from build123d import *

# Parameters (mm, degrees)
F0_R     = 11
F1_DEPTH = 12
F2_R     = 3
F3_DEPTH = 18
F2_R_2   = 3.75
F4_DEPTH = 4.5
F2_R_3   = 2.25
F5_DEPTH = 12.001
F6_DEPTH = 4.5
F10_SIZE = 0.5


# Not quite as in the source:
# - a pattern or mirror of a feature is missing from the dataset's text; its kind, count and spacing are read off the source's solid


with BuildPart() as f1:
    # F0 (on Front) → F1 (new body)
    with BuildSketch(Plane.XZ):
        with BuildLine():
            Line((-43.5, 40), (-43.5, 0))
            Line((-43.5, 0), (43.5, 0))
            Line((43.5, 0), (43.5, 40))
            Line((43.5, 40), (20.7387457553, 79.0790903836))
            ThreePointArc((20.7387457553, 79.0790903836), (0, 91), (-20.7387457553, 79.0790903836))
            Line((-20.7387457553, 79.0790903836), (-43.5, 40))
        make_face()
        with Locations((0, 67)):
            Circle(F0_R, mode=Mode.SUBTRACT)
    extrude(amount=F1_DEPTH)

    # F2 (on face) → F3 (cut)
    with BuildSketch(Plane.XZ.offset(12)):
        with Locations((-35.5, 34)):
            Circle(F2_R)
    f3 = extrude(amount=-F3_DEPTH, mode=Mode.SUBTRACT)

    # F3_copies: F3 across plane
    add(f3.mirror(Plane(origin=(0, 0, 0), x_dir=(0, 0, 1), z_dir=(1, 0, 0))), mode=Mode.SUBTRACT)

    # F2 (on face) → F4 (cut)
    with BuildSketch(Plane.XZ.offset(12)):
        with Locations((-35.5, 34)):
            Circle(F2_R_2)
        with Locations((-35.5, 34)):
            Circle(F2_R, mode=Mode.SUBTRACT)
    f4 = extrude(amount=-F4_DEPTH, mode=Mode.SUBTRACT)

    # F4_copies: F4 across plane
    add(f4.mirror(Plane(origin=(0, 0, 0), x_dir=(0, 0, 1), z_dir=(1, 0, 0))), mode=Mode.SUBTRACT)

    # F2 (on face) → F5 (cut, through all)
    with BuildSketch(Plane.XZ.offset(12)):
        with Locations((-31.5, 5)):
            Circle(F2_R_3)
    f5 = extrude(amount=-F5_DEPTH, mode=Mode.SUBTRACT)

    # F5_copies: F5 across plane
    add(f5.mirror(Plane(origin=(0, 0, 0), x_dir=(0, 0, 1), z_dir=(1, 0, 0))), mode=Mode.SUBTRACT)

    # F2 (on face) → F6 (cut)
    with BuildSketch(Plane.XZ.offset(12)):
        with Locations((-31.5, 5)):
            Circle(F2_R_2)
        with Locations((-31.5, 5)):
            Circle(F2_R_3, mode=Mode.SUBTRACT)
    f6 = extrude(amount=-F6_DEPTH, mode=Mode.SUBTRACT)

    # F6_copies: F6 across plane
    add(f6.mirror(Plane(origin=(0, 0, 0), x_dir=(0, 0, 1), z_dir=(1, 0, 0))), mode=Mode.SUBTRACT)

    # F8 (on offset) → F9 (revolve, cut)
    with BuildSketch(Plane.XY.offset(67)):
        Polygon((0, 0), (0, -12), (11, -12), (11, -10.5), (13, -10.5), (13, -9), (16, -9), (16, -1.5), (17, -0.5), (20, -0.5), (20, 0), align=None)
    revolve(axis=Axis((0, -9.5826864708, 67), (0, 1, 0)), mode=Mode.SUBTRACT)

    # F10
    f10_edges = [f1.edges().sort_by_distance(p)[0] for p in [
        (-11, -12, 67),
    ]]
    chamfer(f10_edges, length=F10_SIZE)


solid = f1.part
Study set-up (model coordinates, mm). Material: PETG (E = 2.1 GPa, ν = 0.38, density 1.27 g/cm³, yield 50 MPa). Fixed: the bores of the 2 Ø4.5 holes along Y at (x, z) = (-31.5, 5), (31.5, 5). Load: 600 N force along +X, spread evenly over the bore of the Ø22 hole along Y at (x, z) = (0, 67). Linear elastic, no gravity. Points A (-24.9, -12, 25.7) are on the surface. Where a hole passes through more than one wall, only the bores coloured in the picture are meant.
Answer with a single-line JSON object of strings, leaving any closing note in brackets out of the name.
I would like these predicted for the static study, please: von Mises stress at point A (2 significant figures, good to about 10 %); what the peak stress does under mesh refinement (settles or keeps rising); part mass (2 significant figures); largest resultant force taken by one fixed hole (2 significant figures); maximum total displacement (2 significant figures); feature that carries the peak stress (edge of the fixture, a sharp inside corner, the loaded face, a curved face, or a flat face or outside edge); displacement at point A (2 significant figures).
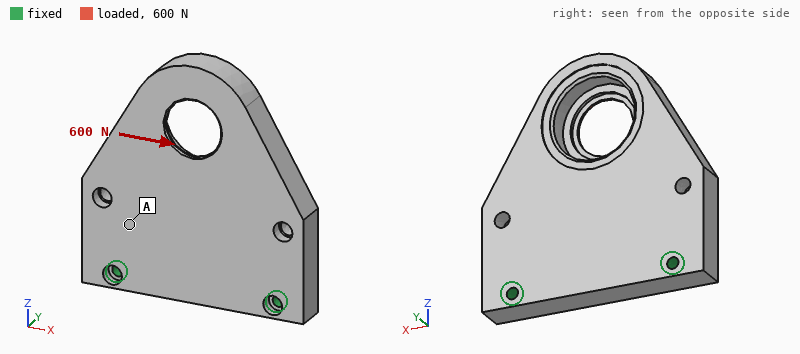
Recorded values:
{"von Mises stress at point A": "1.7 MPa", "what the peak stress does under mesh refinement": "keeps rising", "part mass": "83 g", "largest resultant force taken by one fixed hole": "650 N", "maximum total displacement": "0.27 mm", "feature that carries the peak stress": "edge of the fixture", "displacement at point A": "0.050 mm"}
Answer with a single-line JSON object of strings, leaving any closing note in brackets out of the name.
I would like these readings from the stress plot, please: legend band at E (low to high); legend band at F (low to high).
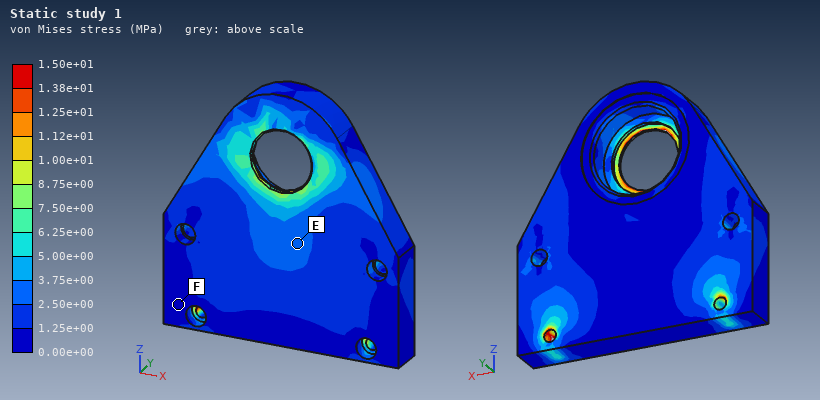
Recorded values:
{"legend band at E": "2.50e+00 to 3.75e+00 MPa", "legend band at F": "0.00e+00 to 1.25e+00 MPa"}
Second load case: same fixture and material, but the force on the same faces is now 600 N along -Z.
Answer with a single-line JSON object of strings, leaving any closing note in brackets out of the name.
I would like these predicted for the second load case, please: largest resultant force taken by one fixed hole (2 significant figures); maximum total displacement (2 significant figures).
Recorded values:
{"largest resultant force taken by one fixed hole": "310 N", "maximum total displacement": "1.0 mm"}
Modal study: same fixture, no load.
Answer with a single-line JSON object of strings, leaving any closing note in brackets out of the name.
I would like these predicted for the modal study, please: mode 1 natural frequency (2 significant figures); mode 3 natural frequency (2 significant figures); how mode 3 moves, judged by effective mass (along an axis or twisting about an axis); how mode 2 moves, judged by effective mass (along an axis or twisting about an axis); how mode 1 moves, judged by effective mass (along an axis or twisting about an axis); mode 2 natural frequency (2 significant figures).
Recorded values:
{"mode 1 natural frequency": "320 Hz", "mode 3 natural frequency": "1600 Hz", "how mode 3 moves, judged by effective mass": "along Y", "how mode 2 moves, judged by effective mass": "twisting about Z", "how mode 1 moves, judged by effective mass": "along Y", "mode 2 natural frequency": "1100 Hz"}
